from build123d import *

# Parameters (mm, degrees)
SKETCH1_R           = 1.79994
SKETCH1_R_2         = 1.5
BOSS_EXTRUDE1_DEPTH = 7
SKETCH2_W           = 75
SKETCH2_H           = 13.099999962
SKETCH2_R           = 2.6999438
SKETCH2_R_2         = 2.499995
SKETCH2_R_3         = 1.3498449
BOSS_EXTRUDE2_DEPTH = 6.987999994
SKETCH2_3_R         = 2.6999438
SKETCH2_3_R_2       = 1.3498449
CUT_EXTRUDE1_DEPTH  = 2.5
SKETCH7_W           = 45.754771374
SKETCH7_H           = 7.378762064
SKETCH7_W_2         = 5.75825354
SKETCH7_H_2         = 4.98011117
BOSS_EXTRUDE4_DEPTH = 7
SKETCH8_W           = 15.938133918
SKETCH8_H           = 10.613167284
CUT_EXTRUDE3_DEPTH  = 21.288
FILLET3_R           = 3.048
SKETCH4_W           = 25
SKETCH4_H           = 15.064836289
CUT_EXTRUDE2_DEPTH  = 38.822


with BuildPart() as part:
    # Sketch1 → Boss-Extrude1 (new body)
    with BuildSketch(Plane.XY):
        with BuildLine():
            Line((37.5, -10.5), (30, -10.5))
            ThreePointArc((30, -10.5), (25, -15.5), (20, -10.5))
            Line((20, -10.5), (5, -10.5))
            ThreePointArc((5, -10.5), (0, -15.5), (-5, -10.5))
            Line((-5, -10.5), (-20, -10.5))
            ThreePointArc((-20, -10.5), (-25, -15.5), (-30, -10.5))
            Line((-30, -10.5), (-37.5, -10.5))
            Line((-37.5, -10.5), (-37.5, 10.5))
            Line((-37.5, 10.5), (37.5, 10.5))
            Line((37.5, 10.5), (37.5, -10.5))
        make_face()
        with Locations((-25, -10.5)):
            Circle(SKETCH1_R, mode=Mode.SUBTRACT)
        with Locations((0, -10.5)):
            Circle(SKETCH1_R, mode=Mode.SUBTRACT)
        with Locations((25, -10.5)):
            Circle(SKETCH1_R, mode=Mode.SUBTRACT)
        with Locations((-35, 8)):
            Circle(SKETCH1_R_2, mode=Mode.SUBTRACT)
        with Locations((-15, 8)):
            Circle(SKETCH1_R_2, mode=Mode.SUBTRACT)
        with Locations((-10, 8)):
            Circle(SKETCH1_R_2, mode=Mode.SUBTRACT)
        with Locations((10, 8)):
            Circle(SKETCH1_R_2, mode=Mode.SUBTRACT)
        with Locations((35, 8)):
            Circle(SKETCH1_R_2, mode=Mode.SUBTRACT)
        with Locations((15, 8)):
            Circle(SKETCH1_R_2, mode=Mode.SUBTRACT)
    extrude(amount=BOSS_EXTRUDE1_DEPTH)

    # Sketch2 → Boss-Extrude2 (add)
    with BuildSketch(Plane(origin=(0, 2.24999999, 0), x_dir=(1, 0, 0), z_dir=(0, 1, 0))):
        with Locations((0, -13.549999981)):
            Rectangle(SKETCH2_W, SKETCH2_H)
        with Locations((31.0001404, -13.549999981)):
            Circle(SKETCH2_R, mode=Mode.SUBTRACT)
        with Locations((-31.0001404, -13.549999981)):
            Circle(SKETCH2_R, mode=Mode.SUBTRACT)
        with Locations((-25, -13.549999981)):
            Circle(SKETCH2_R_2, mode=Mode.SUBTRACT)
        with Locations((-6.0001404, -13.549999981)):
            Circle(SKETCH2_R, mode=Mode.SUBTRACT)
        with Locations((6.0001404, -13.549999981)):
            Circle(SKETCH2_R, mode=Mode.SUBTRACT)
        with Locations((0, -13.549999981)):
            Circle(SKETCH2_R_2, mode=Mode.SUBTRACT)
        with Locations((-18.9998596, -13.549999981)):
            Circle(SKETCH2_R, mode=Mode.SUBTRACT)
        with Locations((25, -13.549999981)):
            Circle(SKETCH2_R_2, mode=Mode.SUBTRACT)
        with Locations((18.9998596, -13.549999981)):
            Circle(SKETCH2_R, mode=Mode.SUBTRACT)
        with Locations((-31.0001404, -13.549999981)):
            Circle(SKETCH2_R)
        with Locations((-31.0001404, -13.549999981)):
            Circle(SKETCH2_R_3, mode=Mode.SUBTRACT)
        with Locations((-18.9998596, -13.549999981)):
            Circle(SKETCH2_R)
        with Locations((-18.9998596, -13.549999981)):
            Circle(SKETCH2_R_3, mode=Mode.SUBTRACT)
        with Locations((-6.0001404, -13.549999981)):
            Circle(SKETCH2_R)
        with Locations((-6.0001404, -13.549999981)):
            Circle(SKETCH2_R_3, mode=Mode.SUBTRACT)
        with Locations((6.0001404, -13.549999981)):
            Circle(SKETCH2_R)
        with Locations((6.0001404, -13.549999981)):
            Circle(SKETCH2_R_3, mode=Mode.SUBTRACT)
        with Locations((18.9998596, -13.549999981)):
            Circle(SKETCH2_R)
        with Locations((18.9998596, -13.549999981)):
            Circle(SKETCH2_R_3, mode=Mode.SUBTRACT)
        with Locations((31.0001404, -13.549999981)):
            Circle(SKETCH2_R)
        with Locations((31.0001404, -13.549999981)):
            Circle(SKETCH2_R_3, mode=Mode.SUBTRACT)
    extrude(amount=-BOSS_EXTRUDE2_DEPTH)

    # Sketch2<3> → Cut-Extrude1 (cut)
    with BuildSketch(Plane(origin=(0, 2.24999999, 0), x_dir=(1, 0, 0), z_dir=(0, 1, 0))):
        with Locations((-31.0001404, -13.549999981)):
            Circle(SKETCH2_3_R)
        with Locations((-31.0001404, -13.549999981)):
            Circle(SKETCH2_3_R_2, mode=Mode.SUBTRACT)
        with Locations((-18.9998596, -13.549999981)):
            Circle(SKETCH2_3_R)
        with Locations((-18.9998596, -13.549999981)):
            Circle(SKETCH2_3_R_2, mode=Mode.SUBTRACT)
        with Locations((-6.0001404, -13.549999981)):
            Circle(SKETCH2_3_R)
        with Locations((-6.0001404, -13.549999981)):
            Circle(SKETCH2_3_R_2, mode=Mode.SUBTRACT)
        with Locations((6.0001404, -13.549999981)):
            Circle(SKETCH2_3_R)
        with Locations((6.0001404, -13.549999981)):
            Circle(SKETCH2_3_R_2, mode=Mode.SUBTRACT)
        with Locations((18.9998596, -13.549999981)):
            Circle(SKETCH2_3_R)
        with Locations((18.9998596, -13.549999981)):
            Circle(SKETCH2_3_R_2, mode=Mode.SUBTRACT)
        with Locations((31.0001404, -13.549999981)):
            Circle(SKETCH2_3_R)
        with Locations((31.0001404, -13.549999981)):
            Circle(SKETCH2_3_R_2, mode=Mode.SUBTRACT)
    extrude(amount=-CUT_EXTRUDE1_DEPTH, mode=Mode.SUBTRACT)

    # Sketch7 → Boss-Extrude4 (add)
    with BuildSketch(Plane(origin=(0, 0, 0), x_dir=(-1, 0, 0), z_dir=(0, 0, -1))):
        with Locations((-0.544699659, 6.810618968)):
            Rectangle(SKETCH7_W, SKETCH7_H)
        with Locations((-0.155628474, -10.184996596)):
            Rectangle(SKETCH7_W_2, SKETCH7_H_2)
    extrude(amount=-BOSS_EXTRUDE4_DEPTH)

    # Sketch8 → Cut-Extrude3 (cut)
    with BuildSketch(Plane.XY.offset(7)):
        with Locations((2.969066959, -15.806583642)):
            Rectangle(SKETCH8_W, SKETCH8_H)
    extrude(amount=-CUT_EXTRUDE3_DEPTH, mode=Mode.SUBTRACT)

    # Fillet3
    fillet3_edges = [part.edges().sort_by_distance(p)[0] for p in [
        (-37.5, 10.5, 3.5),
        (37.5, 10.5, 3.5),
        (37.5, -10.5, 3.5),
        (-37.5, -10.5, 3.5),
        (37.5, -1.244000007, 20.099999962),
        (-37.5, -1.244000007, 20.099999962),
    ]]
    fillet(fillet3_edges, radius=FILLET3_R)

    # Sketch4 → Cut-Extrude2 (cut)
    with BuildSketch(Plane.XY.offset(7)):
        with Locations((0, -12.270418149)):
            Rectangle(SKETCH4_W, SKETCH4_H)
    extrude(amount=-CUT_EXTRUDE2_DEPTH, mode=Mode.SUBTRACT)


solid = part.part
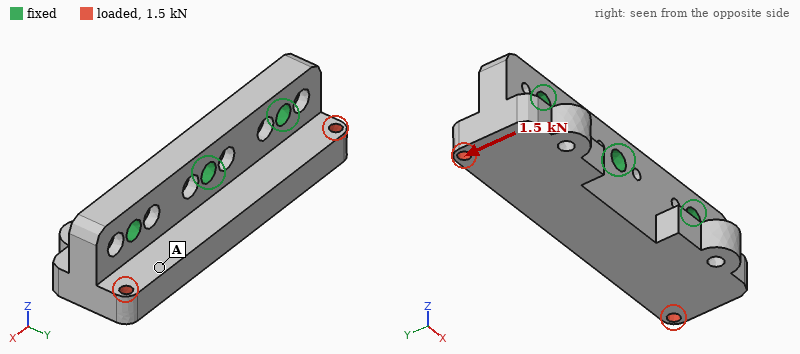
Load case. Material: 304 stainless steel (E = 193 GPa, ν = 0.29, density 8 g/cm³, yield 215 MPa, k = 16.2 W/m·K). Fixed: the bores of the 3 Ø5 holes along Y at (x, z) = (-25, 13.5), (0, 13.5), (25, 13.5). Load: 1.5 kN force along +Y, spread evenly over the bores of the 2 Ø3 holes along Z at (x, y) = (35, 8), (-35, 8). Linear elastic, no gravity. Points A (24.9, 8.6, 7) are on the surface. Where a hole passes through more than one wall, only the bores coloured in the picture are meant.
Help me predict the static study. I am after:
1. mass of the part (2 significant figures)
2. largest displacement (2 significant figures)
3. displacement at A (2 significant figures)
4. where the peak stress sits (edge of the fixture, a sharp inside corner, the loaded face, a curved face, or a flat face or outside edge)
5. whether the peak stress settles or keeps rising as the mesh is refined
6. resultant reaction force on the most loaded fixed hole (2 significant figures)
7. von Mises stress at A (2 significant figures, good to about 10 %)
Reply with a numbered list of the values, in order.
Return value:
1. 130 g
2. 8.7 µm
3. 3.7 µm
4. edge of the fixture
5. keeps rising
6. 840 N
7. 9.9 MPa
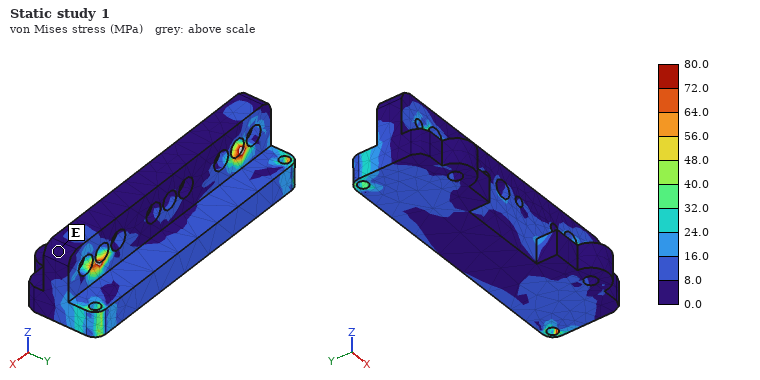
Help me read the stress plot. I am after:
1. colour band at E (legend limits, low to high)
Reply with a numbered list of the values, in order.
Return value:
1. 0.0 to 8.0 MPa
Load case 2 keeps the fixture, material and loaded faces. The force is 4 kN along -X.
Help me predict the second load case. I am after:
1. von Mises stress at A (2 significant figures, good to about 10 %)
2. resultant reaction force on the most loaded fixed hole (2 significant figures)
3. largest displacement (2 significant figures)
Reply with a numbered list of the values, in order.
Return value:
1. 33 MPa
2. 1.6 kN
3. 11 µm
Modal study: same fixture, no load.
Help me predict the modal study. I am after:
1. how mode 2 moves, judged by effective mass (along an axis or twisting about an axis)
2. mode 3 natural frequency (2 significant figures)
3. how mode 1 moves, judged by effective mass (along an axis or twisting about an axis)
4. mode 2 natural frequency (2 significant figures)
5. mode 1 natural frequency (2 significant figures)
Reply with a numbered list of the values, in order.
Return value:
1. twisting about Z
2. 19 kHz
3. along Y
4. 13 kHz
5. 11 kHz
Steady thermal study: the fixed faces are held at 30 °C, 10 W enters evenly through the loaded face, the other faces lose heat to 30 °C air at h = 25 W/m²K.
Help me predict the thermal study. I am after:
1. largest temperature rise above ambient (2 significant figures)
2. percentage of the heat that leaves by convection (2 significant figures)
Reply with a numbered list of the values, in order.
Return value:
1. 65 K
2. 18 %
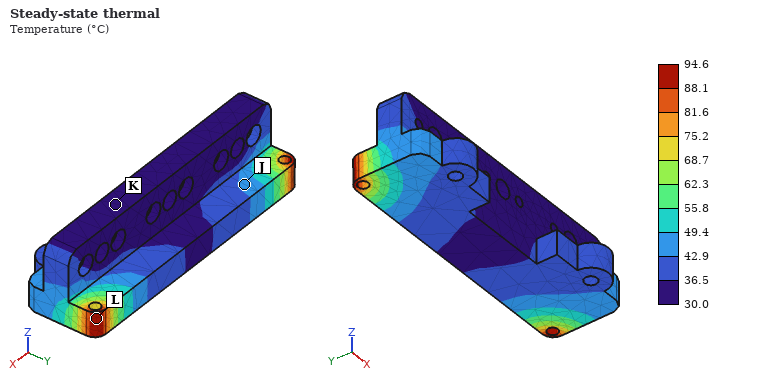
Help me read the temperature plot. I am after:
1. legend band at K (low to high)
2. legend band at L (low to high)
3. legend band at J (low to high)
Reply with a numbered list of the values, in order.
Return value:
1. 30.0 to 36.5 °C
2. 88.1 to 94.6 °C
3. 42.9 to 49.4 °C
